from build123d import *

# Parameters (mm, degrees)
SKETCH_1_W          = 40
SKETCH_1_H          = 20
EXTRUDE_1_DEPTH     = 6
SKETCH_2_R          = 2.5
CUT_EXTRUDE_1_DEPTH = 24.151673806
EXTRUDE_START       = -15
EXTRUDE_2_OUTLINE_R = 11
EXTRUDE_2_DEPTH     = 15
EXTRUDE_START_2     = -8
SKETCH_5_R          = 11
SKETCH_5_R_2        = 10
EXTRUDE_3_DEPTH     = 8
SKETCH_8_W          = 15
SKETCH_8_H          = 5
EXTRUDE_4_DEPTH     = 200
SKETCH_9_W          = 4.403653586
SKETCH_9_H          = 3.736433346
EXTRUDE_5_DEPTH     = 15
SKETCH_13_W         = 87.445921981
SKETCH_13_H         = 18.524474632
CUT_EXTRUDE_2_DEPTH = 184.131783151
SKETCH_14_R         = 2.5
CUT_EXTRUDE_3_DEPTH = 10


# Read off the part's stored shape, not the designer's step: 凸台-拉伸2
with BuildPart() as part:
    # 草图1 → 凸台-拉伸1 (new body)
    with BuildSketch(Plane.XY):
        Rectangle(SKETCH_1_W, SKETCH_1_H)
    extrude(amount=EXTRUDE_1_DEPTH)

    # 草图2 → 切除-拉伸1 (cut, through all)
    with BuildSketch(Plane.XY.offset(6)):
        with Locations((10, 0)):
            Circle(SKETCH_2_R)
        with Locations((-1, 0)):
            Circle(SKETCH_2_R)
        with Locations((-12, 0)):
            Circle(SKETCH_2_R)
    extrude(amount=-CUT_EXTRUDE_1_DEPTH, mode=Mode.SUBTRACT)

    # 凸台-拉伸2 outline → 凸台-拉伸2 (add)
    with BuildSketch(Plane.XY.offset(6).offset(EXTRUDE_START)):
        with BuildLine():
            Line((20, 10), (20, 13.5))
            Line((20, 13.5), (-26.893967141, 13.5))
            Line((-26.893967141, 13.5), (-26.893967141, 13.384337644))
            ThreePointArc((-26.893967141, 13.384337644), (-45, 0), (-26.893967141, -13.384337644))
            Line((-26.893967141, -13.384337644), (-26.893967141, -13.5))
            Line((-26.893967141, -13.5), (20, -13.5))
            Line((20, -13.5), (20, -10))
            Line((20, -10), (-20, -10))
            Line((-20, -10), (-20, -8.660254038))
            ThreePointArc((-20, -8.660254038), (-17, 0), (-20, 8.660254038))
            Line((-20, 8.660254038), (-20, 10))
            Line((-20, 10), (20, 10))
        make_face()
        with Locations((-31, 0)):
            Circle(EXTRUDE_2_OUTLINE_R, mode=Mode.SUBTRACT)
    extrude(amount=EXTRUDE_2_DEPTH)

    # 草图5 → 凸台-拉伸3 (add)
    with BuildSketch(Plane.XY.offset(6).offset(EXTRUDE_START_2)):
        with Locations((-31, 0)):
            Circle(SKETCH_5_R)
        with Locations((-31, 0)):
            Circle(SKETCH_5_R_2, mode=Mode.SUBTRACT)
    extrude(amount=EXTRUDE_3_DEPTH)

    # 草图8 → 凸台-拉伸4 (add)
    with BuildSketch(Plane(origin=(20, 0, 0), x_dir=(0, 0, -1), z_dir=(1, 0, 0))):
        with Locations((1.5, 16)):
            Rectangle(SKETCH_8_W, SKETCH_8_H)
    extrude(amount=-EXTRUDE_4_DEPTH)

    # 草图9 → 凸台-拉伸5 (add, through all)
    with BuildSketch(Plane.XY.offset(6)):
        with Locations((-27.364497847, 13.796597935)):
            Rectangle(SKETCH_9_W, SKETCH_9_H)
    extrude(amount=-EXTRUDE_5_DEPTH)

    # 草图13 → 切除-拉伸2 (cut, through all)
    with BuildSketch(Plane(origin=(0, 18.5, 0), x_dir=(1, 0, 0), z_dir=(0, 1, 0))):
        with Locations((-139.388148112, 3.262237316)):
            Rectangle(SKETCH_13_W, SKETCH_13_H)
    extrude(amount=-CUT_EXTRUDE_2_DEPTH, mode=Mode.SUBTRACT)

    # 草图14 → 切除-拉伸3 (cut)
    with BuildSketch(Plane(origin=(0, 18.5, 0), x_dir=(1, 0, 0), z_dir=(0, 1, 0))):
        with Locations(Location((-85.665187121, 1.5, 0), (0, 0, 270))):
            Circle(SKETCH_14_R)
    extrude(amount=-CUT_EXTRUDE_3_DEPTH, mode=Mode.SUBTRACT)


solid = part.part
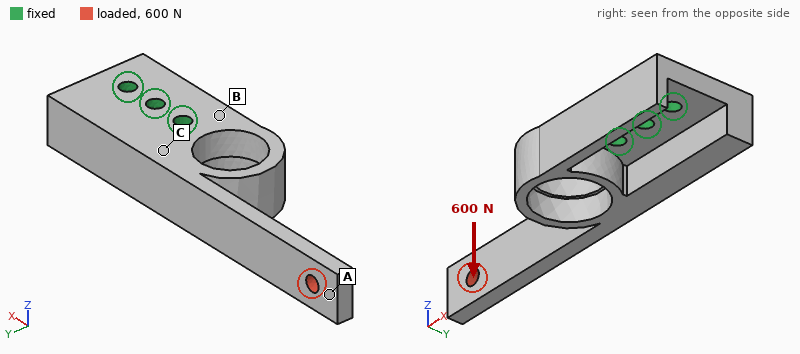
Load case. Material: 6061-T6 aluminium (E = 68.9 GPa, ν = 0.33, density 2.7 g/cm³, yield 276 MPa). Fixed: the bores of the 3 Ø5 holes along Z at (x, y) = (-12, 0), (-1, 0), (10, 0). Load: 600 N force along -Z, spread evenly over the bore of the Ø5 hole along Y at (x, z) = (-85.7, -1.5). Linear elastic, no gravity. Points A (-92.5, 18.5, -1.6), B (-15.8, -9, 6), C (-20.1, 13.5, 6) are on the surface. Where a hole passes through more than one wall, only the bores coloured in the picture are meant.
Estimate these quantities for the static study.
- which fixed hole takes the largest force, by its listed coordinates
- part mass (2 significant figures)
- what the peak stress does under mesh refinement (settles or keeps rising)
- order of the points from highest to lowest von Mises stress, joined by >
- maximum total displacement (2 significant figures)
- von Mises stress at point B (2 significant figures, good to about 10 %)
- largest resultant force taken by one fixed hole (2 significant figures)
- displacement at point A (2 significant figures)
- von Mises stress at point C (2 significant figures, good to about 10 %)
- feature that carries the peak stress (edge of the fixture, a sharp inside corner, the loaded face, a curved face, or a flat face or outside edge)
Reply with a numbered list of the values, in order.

1. (-12, 0)
2. 58 g
3. keeps rising
4. C > B > A
5. 0.93 mm
6. 33 MPa
7. 2.2 kN
8. 0.87 mm
9. 83 MPa
10. edge of the fixture
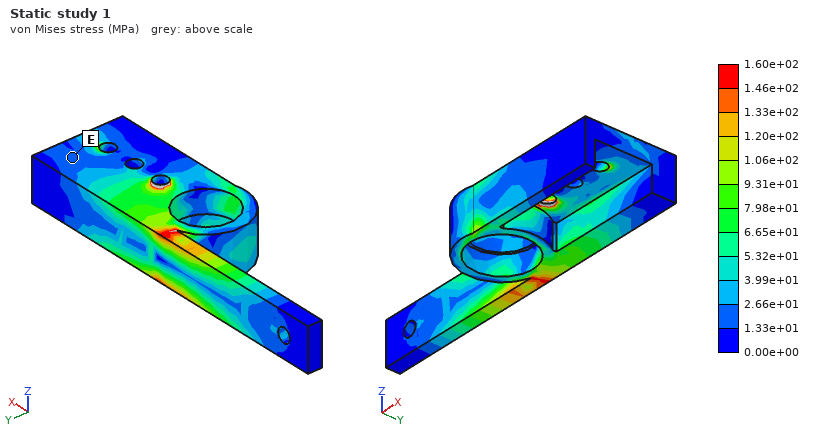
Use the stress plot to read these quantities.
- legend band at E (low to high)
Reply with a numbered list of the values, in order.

1. 1.33e+01 to 2.66e+01 MPa
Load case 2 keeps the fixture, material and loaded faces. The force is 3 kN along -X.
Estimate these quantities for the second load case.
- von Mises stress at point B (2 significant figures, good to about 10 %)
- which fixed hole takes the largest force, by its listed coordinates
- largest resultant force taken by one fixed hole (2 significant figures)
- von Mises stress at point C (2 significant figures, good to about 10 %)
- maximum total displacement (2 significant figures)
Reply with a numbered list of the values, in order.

1. 10.0 MPa
2. (-12, 0)
3. 2.2 kN
4. 21 MPa
5. 0.17 mm
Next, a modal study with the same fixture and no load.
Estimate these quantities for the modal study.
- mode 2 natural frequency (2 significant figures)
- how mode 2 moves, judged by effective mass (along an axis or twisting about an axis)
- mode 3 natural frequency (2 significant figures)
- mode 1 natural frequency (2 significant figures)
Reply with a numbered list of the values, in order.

1. 1800 Hz
2. along Z
3. 5200 Hz
4. 970 Hz
